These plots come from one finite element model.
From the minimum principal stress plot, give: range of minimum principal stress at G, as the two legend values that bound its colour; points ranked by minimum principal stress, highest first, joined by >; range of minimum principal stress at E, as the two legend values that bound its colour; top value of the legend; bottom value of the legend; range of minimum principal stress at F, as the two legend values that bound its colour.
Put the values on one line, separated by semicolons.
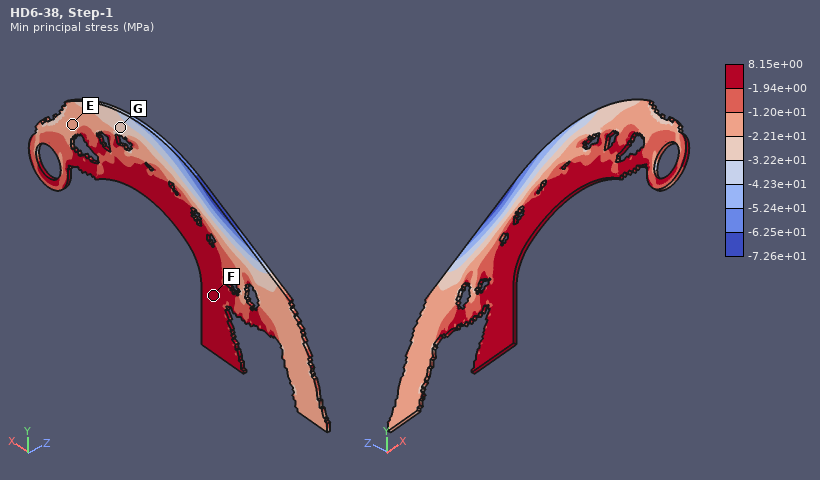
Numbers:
-3.22e+01 to -2.21e+01 MPa; F > E > G; -2.21e+01 to -1.20e+01 MPa; 8.15e+00 MPa; -7.26e+01 MPa; -1.94e+00 to 8.15e+00 MPa
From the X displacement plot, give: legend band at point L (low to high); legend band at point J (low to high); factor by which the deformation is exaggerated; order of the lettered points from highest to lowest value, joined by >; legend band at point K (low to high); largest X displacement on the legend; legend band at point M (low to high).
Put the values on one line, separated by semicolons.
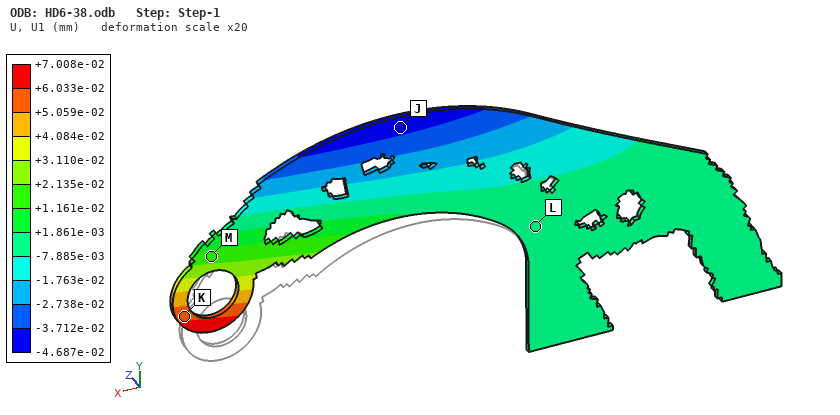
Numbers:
-7.885e-03 to +1.861e-03 mm; -4.687e-02 to -3.712e-02 mm; 20; K > M > L > J; +5.059e-02 to +6.033e-02 mm; +7.008e-02 mm; +1.161e-02 to +2.135e-02 mm
